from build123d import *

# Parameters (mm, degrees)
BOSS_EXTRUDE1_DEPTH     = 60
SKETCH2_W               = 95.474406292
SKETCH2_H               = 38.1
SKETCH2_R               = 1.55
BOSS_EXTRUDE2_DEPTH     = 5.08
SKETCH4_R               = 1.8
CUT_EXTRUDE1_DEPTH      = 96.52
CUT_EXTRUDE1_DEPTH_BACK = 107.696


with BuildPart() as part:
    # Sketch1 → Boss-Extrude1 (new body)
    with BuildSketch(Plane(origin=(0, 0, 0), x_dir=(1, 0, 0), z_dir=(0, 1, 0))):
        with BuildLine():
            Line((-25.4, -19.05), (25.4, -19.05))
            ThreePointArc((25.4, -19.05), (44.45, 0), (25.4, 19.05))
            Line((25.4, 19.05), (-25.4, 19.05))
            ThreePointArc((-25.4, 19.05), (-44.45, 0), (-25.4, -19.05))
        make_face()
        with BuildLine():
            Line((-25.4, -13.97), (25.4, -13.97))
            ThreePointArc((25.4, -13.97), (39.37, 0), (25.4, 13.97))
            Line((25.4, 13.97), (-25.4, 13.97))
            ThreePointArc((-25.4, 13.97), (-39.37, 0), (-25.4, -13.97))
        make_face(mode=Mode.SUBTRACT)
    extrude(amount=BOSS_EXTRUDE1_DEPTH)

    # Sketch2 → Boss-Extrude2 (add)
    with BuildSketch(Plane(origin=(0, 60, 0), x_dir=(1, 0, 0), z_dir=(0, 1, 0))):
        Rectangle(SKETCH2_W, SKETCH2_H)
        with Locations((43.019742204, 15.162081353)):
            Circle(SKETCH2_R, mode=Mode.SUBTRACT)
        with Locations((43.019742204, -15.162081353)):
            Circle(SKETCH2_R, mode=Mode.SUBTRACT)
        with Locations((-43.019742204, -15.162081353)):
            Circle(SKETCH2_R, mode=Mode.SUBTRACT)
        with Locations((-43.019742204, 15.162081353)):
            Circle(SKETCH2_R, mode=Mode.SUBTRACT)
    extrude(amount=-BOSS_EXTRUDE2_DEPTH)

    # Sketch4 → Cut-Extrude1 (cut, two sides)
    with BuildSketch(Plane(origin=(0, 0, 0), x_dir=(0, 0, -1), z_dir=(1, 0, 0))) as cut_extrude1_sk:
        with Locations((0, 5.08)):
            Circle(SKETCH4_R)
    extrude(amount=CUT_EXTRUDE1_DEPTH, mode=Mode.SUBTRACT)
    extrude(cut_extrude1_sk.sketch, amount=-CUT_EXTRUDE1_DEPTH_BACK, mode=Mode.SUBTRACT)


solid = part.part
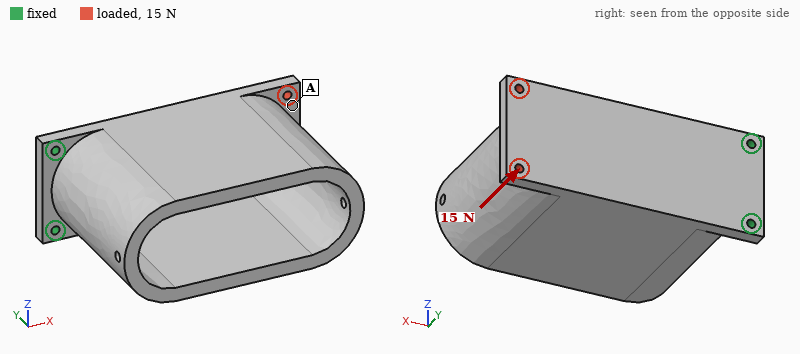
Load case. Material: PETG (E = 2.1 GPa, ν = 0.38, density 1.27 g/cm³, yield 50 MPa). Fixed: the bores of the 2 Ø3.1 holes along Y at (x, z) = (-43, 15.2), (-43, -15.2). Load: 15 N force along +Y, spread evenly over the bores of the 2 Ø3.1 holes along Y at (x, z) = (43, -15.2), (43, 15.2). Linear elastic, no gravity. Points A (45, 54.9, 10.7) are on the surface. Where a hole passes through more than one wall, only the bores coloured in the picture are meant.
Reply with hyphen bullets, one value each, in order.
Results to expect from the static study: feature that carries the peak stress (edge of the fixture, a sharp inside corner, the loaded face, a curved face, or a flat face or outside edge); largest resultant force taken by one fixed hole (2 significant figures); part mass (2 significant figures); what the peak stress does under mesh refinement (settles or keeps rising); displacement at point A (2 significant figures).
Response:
- edge of the fixture
- 10 N
- 96 g
- keeps rising
- 1.0 mm
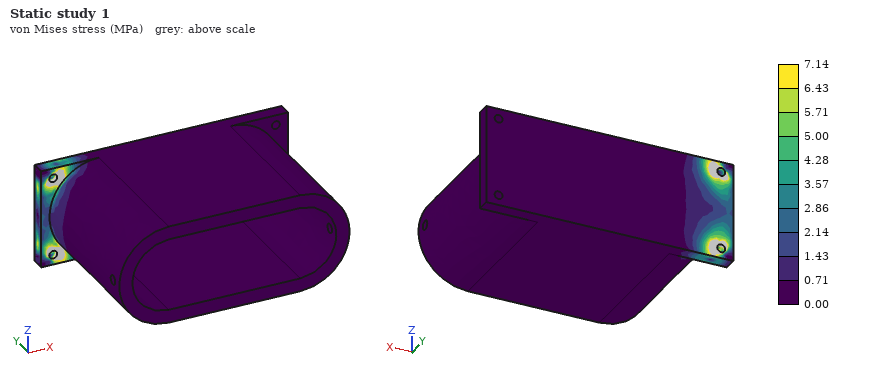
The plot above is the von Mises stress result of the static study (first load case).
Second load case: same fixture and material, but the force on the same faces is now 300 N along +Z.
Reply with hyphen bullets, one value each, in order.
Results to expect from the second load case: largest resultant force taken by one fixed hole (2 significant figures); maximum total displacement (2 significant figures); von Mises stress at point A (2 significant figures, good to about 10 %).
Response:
- 850 N
- 1.2 mm
- 3.2 MPa
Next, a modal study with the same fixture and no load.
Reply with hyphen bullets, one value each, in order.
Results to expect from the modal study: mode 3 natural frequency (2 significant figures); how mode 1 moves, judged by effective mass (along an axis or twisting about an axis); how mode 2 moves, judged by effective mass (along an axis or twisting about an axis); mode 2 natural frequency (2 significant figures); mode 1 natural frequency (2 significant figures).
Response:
- 650 Hz
- along Y
- along Z
- 340 Hz
- 92 Hz
